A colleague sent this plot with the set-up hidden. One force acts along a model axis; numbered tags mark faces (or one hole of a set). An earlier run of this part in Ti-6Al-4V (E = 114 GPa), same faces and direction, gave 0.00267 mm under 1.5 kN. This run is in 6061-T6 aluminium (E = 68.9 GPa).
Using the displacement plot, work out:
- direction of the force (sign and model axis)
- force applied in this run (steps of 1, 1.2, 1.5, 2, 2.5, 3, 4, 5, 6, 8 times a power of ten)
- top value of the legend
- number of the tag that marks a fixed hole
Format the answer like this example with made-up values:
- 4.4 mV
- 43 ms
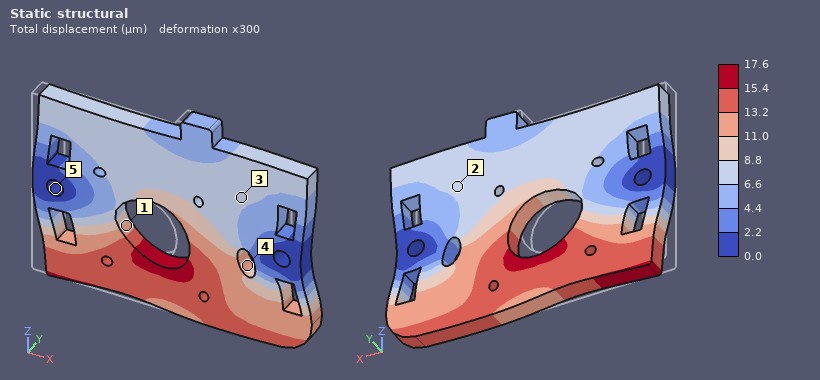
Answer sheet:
- +X
- 6 kN
- 17.6 µm
- 5
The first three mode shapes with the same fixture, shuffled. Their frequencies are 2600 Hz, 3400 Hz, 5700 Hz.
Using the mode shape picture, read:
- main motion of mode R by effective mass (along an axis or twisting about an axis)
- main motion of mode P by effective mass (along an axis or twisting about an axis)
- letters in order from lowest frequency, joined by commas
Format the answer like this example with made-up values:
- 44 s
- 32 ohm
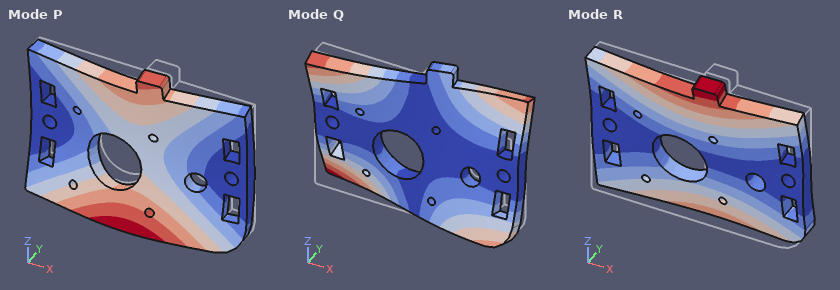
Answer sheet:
- twisting about X
- along Y
- R, P, Q
